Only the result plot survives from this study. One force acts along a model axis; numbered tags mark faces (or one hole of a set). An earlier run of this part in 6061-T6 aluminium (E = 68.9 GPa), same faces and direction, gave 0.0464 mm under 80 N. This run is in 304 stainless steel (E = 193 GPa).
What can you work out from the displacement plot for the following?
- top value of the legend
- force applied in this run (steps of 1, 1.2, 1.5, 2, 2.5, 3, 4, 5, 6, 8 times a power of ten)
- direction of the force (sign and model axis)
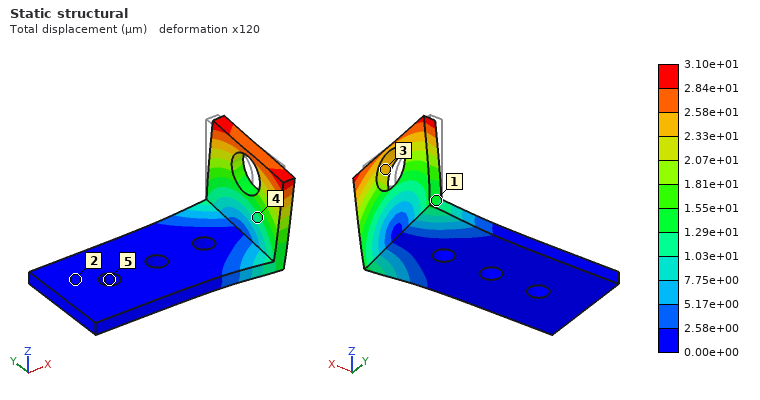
3.10e+01 µm
150 N
-Y
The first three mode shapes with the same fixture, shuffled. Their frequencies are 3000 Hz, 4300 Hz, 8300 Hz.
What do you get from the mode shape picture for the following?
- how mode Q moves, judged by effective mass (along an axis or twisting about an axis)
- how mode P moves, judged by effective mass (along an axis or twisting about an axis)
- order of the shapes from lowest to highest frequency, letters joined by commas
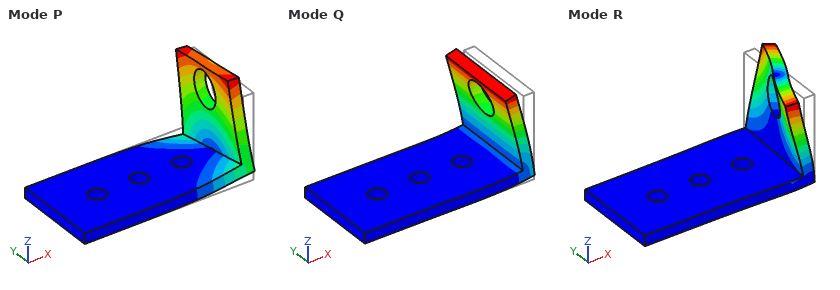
along X
along Y
Q, P, R
